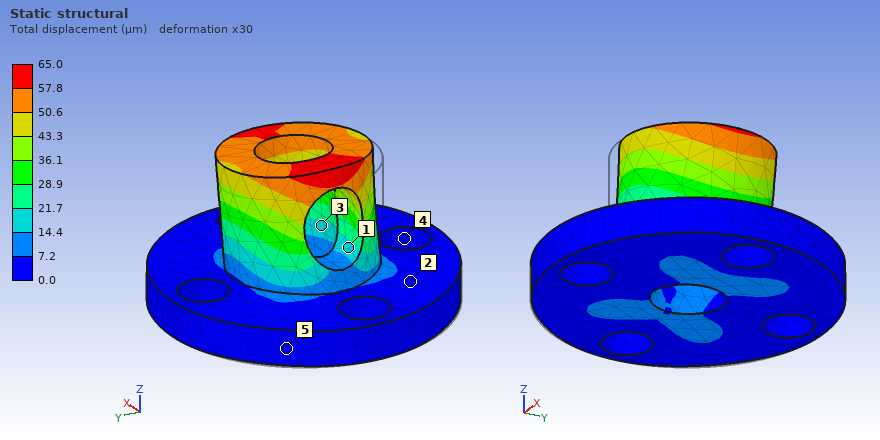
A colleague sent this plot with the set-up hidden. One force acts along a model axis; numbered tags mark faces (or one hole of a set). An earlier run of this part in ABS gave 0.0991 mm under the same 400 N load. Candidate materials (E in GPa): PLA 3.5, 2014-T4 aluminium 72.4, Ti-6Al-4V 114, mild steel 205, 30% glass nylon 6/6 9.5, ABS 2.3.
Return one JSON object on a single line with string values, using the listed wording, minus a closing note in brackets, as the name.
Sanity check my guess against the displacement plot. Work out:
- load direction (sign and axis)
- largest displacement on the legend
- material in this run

{"load direction": "+X", "largest displacement on the legend": "65.0 µm", "material in this run": "PLA"}
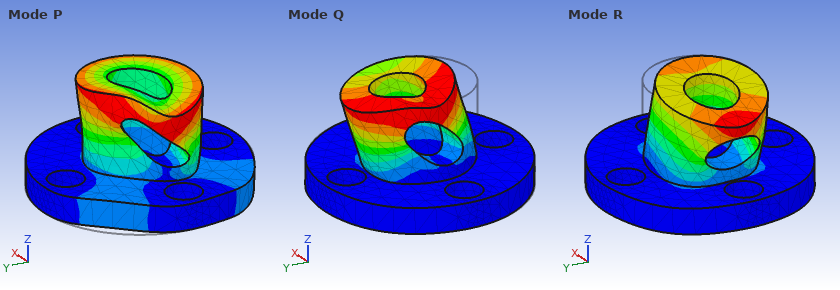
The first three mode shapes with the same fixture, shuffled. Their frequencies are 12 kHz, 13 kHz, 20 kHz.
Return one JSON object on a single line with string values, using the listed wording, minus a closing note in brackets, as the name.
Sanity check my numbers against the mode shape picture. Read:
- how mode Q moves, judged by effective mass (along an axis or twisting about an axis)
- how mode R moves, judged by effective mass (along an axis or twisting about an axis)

{"how mode Q moves, judged by effective mass": "along Y", "how mode R moves, judged by effective mass": "along X"}
